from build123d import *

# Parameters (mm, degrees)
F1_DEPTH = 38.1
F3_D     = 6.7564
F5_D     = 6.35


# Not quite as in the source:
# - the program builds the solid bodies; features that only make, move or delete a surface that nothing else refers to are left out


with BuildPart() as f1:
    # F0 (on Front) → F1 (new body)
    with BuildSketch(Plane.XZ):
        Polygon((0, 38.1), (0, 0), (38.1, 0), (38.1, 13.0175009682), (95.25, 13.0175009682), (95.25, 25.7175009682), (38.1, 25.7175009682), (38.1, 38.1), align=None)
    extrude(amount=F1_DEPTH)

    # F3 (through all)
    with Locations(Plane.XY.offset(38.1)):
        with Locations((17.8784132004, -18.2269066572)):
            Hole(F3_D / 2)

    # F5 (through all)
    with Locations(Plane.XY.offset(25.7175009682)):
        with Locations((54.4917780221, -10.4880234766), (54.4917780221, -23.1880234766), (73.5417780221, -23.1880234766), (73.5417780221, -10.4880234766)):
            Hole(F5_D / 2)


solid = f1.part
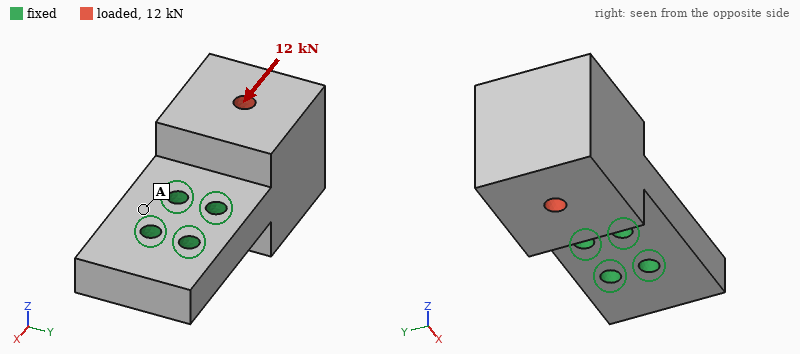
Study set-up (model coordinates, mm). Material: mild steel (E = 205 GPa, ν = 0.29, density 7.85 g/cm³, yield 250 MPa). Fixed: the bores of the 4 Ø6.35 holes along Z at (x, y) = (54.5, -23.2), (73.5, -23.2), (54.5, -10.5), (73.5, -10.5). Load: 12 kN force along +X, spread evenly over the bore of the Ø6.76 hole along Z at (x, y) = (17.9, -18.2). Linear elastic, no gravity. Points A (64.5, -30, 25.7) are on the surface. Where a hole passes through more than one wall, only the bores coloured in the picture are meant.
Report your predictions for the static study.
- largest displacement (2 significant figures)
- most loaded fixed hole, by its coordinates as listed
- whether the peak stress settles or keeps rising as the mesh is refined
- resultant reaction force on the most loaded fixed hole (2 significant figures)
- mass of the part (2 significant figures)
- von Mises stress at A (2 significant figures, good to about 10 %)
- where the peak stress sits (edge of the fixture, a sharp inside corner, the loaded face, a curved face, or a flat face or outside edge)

5.7 µm
(54.5, -23.2)
keeps rising
5.7 kN
630 g
8.6 MPa
edge of the fixture
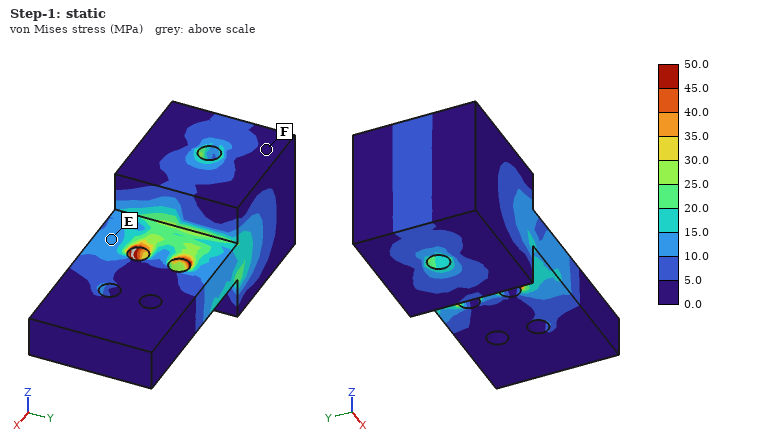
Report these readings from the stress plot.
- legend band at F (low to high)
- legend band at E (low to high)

0.0 to 5.0 MPa
10.0 to 15.0 MPa
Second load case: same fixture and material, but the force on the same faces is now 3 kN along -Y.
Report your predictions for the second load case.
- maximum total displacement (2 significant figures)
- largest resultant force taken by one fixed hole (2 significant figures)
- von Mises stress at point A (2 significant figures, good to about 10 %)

13 µm
4.4 kN
13 MPa
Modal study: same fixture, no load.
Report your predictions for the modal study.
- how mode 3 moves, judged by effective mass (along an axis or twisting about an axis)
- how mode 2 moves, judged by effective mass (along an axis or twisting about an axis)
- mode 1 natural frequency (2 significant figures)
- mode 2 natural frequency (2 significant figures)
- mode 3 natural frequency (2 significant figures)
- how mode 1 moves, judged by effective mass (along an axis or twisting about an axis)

twisting about X
along Y
2100 Hz
4400 Hz
5800 Hz
along Z
